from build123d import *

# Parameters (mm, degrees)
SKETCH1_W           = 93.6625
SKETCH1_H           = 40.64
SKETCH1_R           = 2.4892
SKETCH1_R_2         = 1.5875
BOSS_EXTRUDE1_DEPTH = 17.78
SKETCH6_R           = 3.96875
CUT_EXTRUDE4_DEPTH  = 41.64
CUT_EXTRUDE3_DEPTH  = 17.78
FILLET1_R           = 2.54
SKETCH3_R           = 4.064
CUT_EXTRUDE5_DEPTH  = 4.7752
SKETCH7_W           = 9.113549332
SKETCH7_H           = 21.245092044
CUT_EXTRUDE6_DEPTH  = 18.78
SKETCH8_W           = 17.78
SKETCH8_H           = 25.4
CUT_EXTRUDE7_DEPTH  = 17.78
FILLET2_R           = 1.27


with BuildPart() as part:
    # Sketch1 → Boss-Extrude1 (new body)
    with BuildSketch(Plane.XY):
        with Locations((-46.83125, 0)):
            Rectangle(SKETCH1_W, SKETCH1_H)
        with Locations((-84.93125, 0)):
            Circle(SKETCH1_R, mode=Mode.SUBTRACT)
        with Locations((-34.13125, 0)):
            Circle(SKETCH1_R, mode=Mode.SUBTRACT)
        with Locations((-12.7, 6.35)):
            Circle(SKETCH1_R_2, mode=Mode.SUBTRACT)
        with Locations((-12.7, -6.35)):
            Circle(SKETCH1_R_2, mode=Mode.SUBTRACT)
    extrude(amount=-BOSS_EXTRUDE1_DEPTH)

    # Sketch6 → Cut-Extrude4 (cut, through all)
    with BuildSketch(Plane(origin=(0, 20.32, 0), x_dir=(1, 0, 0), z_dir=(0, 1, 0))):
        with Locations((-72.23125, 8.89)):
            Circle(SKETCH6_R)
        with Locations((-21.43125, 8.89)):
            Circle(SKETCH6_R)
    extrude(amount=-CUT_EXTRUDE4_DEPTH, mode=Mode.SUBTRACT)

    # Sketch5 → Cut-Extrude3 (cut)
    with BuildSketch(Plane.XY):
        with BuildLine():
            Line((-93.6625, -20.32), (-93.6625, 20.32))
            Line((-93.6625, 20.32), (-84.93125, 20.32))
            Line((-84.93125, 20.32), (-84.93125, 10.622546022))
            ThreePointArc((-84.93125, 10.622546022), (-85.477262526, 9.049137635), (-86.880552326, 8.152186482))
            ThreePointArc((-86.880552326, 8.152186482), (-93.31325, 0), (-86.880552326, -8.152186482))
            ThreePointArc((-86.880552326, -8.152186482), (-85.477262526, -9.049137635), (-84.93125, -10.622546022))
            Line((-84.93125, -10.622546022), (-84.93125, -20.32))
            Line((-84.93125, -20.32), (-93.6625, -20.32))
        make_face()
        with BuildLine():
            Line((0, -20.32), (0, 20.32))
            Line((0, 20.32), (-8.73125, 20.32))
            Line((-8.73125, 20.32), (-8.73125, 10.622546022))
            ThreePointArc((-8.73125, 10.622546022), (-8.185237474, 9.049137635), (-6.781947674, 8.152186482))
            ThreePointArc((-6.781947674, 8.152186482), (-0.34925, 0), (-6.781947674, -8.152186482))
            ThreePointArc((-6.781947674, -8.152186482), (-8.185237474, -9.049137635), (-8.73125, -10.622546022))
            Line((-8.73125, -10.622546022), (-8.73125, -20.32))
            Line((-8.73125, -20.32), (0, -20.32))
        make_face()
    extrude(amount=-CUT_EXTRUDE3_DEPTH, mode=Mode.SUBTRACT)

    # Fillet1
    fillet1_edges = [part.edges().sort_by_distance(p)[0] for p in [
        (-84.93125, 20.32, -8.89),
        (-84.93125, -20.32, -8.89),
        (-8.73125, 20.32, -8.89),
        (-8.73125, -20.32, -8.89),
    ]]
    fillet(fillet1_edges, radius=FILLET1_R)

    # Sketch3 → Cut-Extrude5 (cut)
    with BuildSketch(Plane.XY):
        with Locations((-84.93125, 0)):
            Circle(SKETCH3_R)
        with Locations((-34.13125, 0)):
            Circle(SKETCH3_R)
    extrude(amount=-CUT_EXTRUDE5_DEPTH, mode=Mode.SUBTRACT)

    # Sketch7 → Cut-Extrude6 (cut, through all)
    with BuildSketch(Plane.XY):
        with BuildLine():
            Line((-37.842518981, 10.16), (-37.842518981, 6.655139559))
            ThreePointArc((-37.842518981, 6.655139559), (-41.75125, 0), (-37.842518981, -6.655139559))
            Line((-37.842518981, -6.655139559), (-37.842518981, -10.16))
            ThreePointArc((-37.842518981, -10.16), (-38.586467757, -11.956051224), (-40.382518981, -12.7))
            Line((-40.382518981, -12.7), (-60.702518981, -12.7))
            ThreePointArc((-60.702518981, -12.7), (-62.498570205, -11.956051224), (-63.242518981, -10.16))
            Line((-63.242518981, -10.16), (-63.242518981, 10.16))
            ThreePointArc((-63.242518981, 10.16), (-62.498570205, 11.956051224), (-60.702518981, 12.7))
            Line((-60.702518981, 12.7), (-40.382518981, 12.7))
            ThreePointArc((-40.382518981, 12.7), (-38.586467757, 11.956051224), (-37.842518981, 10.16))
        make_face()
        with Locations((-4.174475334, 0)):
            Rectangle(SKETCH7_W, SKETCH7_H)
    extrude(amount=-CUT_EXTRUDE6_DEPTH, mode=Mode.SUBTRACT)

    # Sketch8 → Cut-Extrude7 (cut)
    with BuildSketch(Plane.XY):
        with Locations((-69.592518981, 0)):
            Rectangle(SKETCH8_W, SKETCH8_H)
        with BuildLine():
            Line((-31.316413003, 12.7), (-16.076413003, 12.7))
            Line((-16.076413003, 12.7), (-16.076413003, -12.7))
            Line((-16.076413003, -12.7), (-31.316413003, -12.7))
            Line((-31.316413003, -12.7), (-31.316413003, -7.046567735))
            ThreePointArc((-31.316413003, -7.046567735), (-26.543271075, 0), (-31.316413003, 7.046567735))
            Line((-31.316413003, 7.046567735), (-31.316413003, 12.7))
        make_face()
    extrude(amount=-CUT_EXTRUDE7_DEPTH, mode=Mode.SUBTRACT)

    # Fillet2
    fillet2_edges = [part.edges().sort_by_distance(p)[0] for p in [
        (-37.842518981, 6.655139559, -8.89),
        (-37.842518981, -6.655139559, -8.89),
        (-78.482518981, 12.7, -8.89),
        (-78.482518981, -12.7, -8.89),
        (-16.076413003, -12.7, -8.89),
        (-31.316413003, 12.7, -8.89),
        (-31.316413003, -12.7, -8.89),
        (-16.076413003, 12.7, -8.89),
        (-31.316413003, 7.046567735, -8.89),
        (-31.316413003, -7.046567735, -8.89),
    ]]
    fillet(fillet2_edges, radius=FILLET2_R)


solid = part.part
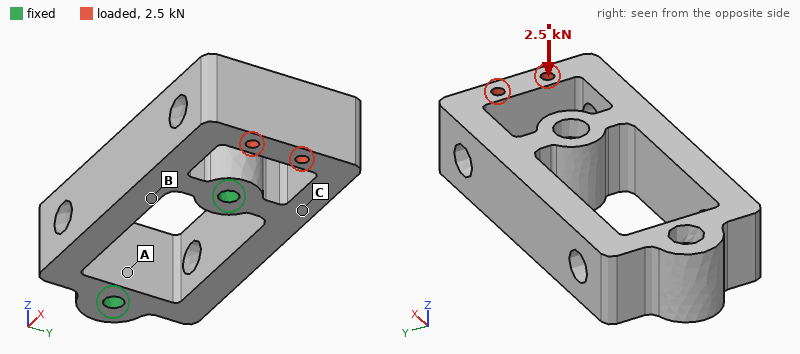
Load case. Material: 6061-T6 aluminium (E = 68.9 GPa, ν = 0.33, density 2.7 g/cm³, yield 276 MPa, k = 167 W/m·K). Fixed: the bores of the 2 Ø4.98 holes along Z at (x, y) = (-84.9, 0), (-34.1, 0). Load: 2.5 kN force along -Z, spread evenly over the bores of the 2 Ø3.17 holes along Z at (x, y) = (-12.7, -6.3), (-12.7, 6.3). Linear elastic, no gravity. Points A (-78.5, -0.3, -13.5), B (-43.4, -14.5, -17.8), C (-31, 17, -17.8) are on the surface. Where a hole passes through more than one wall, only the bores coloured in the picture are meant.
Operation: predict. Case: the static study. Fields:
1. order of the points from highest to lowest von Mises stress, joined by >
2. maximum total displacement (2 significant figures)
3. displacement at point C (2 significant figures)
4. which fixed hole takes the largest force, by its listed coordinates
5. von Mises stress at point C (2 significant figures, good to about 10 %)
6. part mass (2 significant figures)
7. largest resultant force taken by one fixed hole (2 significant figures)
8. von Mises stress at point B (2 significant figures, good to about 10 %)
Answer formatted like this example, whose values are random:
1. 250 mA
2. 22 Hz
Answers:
1. C > B > A
2. 0.11 mm
3. 0.030 mm
4. (-34.1, 0)
5. 64 MPa
6. 82 g
7. 3.3 kN
8. 33 MPa
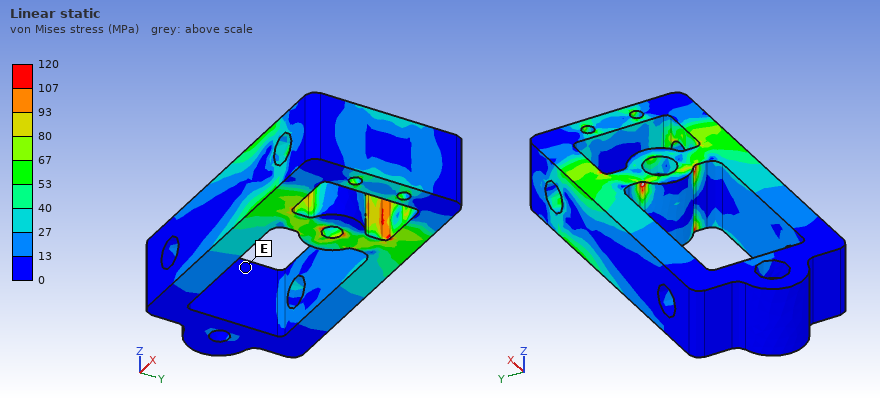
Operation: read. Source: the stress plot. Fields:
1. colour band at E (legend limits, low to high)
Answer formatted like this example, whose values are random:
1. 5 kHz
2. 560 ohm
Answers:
1. 0 to 13 MPa
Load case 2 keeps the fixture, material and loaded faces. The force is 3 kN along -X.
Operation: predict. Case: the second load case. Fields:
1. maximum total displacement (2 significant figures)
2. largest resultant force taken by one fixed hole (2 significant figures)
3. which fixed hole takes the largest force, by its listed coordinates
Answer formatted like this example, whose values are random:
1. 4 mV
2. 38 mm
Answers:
1. 41 µm
2. 1.8 kN
3. (-34.1, 0)
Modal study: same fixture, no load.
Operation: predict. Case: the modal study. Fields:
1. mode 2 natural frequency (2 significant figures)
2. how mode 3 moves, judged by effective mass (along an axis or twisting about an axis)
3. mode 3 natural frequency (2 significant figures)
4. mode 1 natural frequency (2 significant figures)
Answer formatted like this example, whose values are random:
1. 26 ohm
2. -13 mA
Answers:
1. 6400 Hz
2. twisting about X
3. 8400 Hz
4. 6400 Hz
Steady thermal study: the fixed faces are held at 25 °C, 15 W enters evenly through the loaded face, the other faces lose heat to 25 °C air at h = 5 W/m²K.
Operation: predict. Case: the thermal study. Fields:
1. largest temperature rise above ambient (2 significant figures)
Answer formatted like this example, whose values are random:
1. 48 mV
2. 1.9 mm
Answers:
1. 16 K
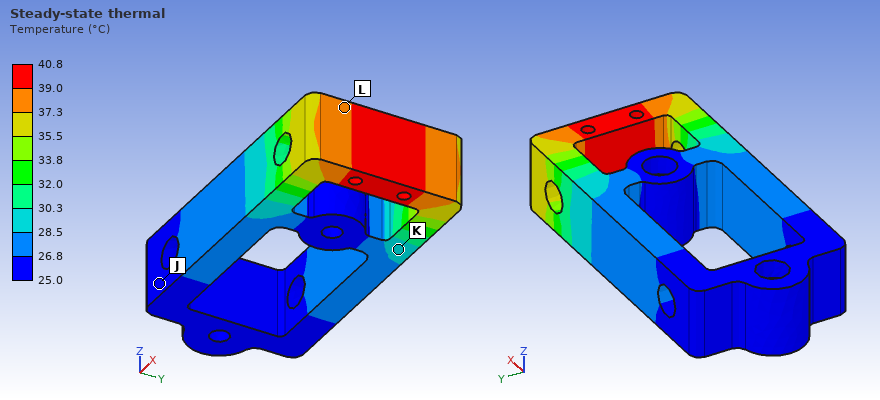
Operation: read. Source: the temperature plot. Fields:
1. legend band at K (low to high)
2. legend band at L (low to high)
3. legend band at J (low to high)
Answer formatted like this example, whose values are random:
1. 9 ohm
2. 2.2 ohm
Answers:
1. 28.5 to 30.3 °C
2. 37.3 to 39.0 °C
3. 25.0 to 26.8 °C
